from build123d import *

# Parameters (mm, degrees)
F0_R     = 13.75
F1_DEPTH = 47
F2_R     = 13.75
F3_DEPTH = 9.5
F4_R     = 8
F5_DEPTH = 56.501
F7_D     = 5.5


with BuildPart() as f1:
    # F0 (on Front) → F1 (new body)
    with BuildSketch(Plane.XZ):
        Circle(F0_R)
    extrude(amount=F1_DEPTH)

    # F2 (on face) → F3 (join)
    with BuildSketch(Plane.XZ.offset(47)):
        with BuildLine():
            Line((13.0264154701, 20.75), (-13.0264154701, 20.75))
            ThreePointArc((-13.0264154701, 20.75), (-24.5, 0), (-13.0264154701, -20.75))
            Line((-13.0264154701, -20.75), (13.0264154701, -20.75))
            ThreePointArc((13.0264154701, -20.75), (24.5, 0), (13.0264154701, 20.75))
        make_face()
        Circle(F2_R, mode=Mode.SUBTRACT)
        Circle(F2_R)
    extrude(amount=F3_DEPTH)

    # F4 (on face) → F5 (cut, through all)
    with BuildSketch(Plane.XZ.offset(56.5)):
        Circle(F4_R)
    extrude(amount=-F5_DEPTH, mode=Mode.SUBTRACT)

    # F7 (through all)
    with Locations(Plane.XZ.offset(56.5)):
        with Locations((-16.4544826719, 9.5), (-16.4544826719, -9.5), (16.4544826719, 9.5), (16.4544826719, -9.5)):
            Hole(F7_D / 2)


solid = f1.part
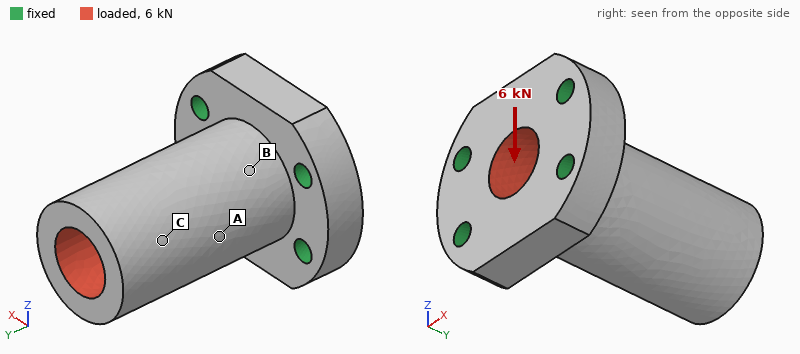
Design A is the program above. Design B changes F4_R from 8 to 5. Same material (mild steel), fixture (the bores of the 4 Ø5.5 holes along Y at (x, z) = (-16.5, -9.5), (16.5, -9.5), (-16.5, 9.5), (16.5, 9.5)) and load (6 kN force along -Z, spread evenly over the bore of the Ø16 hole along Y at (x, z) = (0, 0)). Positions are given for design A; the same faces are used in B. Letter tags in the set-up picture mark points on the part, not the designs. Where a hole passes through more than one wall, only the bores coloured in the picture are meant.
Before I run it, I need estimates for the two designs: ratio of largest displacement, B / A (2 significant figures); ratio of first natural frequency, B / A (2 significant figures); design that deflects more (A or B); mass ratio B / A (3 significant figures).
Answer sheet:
0.88
0.94
A
1.21
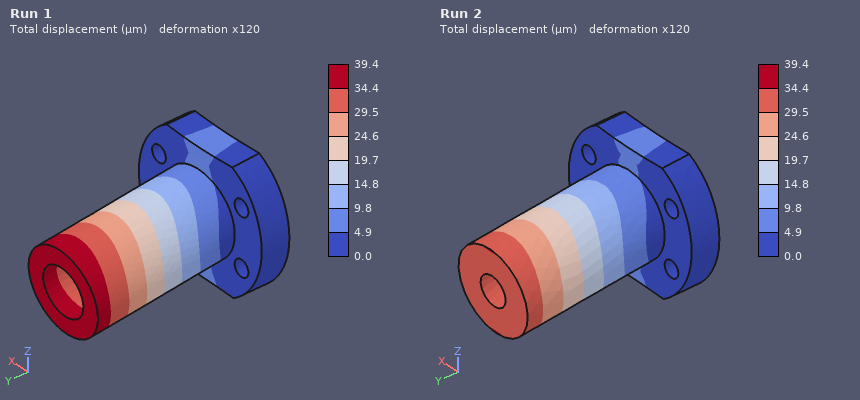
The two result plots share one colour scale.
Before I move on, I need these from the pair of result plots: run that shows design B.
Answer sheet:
Run 2
